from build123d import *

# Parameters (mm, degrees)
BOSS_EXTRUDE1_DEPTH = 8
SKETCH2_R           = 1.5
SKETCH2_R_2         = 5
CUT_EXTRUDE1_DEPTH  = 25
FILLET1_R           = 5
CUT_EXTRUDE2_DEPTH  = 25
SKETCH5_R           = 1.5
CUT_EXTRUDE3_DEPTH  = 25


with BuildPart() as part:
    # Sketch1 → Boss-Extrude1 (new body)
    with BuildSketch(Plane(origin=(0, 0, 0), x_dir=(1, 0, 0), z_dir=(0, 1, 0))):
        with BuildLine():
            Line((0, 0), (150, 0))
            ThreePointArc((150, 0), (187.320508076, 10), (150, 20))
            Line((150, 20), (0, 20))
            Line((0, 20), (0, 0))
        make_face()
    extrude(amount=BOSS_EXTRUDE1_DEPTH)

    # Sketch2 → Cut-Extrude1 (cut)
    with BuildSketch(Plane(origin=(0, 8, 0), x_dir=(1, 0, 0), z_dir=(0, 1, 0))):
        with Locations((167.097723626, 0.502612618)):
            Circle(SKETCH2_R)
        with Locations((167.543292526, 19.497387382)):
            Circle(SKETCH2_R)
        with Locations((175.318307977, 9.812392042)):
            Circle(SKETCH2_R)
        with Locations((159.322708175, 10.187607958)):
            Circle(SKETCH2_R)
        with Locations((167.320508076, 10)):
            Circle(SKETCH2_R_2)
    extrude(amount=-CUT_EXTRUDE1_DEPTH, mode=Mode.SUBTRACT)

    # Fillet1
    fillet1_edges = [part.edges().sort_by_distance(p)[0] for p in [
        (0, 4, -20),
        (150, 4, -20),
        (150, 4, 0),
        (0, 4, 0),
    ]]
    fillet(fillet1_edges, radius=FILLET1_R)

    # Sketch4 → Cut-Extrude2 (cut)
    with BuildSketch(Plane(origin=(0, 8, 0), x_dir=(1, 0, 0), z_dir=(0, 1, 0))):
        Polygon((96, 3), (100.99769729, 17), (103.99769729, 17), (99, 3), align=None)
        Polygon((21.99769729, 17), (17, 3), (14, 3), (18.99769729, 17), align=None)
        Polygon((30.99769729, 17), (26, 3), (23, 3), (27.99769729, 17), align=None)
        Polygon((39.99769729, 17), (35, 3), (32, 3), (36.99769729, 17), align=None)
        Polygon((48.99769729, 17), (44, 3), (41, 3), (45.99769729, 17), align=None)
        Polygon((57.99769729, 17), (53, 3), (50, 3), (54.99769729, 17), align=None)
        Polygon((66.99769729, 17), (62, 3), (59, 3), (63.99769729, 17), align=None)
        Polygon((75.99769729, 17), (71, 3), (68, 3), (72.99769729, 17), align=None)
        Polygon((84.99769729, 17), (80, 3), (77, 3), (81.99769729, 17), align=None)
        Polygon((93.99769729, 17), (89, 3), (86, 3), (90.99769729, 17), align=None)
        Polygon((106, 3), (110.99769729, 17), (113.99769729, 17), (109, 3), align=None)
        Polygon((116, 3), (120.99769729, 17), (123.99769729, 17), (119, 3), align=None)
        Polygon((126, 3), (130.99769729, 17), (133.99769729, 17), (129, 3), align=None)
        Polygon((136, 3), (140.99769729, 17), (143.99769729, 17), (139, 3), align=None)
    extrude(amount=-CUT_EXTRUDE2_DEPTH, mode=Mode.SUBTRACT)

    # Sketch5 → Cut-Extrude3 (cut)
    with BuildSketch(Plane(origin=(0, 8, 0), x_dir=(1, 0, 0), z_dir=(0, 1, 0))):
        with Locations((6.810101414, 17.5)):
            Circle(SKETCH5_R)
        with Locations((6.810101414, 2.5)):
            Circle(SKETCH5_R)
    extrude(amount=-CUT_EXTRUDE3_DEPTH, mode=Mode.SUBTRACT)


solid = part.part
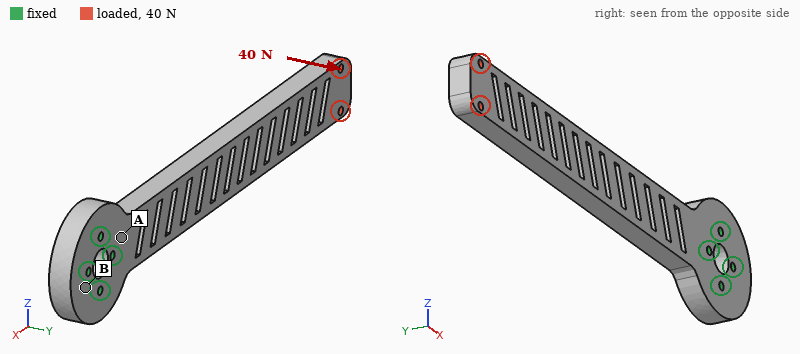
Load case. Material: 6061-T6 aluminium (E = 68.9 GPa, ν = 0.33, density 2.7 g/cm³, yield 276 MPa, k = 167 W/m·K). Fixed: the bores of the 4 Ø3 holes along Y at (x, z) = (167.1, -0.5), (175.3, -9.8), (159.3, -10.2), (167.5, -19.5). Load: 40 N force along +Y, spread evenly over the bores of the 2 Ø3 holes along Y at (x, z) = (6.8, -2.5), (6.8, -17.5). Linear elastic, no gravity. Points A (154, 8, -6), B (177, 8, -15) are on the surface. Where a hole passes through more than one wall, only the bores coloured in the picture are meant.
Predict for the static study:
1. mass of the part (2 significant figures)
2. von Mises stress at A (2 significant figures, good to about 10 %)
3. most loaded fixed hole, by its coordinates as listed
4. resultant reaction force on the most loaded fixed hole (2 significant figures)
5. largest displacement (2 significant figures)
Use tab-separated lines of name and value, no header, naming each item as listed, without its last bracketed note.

mass of the part	76 g
von Mises stress at A	20 MPa
most loaded fixed hole, by its coordinates as listed	(159.3, -10.2)
resultant reaction force on the most loaded fixed hole	270 N
largest displacement	2.0 mm
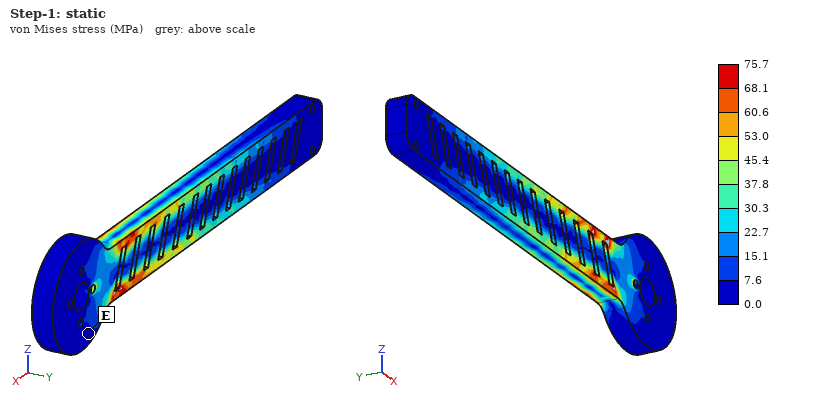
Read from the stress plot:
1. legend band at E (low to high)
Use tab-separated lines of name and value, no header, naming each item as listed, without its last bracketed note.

legend band at E	0.0 to 7.6 MPa
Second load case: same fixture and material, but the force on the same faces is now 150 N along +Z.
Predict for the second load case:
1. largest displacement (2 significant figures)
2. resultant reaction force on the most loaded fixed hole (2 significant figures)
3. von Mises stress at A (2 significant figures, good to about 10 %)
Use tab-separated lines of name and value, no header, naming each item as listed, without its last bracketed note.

largest displacement	0.69 mm
resultant reaction force on the most loaded fixed hole	1.0 kN
von Mises stress at A	11 MPa
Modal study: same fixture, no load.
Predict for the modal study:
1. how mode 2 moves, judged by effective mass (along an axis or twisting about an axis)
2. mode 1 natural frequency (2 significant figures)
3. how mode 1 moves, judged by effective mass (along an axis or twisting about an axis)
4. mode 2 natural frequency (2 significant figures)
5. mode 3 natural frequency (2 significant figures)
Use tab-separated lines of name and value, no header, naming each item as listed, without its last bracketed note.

how mode 2 moves, judged by effective mass	along Z
mode 1 natural frequency	190 Hz
how mode 1 moves, judged by effective mass	along Y
mode 2 natural frequency	620 Hz
mode 3 natural frequency	1200 Hz
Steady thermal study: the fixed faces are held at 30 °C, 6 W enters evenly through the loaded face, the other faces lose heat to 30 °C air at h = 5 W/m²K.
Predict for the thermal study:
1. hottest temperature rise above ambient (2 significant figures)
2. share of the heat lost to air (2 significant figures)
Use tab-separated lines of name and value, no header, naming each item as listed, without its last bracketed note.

hottest temperature rise above ambient	65 K
share of the heat lost to air	31 %
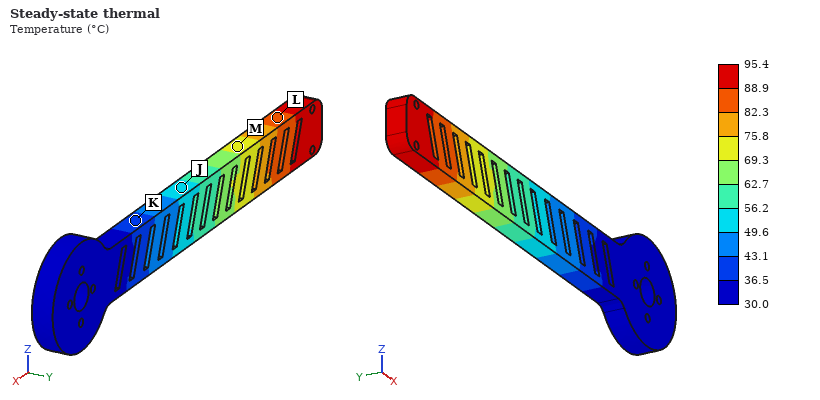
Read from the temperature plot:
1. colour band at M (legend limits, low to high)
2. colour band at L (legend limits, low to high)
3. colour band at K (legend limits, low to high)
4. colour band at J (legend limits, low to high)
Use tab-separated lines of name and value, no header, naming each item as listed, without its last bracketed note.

colour band at M	69.3 to 75.8 °C
colour band at L	82.3 to 88.9 °C
colour band at K	36.5 to 43.1 °C
colour band at J	49.6 to 56.2 °C
